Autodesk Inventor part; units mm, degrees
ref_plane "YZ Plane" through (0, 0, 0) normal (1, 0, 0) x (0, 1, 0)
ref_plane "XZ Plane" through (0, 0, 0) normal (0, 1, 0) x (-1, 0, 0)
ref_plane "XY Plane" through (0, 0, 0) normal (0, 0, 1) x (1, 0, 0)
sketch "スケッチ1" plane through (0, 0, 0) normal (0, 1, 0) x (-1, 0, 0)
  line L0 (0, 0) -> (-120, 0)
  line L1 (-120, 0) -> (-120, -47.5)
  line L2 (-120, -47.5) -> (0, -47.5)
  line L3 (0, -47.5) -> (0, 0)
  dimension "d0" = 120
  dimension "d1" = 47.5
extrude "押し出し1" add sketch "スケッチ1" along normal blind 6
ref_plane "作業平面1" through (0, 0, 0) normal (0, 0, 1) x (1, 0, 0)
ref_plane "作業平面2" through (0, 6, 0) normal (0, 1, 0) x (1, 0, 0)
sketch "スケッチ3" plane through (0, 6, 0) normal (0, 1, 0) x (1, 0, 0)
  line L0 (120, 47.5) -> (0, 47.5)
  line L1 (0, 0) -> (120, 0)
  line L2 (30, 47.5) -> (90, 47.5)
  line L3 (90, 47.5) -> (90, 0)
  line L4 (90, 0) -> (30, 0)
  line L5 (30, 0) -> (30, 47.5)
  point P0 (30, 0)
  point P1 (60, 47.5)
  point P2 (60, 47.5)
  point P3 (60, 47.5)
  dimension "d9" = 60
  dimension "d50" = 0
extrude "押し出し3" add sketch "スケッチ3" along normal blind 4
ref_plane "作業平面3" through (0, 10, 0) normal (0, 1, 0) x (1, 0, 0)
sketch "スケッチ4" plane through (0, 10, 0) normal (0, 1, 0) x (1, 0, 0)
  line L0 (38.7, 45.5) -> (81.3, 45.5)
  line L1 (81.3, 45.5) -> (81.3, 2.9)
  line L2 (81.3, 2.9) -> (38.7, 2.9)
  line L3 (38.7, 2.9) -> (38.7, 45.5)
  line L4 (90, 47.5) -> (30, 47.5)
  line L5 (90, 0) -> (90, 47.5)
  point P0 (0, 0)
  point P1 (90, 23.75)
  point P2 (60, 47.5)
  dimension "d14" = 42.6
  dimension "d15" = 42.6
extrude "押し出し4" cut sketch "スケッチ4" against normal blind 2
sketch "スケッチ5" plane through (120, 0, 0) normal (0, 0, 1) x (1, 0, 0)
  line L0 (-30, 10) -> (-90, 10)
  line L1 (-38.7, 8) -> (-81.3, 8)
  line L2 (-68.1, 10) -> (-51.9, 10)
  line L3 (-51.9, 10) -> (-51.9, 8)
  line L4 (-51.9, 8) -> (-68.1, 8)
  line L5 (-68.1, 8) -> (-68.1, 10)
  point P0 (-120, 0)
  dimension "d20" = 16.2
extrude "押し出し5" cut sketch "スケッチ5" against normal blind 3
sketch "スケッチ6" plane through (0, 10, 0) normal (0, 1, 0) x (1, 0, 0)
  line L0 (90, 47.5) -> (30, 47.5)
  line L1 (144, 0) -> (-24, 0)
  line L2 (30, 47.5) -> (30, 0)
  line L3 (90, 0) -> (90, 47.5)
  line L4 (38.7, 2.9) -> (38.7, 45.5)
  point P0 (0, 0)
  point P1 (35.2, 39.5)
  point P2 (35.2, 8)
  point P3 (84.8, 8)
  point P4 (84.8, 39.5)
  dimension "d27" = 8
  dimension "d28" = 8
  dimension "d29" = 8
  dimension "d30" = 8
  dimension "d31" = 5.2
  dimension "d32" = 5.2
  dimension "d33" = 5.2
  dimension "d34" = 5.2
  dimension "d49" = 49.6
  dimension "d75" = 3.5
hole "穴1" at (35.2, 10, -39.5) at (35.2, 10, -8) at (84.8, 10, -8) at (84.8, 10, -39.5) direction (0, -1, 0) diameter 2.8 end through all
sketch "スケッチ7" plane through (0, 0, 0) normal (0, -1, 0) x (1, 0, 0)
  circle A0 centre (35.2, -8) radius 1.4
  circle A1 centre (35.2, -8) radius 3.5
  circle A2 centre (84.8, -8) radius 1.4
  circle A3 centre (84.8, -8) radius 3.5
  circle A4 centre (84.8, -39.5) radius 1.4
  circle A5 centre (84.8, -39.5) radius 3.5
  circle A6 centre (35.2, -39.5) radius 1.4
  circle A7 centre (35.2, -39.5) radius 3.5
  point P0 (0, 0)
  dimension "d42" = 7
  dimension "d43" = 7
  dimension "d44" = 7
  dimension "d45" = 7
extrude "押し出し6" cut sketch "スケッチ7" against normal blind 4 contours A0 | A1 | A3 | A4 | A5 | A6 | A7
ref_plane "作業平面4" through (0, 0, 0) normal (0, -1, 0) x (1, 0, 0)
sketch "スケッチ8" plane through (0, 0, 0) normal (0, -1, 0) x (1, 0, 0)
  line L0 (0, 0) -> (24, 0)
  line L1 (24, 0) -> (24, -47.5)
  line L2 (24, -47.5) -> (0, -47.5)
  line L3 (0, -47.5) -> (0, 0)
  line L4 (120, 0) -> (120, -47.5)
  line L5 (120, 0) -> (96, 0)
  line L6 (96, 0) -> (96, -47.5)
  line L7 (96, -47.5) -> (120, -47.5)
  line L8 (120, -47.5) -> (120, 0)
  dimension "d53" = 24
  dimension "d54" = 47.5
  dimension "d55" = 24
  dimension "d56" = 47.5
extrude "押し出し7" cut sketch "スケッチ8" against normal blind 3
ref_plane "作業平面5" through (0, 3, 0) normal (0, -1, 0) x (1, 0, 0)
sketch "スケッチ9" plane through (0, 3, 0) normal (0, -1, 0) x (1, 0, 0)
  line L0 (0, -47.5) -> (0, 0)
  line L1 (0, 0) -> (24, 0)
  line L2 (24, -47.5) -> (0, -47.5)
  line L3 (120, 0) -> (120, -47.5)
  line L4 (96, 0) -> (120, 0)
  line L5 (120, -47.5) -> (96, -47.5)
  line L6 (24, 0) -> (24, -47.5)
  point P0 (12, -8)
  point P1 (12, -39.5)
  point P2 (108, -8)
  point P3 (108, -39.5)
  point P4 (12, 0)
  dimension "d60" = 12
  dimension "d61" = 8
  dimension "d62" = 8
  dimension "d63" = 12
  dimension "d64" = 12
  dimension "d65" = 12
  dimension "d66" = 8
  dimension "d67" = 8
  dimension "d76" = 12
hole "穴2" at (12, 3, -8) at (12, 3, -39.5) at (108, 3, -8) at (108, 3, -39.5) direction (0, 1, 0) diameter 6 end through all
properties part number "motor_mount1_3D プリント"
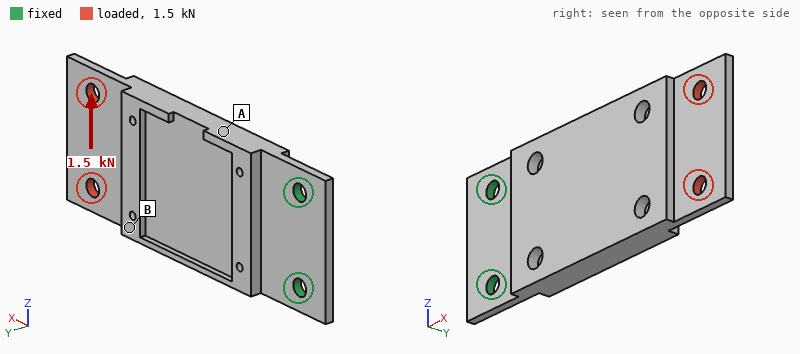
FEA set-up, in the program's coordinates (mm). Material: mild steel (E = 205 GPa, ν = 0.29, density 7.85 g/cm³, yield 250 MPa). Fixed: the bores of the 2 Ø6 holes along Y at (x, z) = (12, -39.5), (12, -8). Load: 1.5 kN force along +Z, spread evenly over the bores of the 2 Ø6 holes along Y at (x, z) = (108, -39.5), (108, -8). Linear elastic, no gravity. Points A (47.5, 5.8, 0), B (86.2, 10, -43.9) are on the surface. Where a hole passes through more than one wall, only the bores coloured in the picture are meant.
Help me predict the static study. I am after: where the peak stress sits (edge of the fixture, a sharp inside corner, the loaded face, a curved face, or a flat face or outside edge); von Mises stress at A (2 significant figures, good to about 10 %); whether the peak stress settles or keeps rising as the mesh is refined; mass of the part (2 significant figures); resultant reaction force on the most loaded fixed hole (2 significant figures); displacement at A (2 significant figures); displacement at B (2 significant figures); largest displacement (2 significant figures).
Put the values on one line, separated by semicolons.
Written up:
edge of the fixture; 31 MPa; keeps rising; 270 g; 4.3 kN; 23 µm; 50 µm; 78 µm
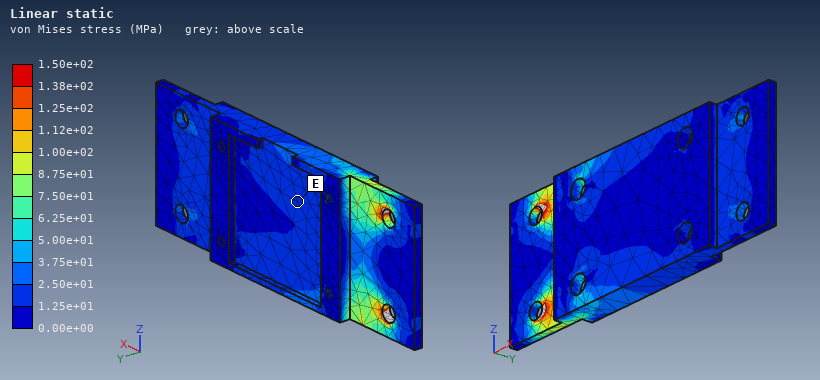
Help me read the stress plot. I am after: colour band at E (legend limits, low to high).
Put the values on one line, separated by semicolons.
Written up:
1.25e+01 to 2.50e+01 MPa
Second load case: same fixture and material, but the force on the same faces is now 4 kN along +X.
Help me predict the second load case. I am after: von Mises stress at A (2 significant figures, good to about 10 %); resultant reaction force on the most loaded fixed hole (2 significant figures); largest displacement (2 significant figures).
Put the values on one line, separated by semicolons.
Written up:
12 MPa; 2.0 kN; 38 µm
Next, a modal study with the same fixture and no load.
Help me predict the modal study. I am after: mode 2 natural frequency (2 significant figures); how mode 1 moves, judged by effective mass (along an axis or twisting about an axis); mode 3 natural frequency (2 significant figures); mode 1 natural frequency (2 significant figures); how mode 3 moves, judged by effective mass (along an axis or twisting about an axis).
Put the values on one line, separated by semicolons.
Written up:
2200 Hz; along Y; 2700 Hz; 260 Hz; along Z
